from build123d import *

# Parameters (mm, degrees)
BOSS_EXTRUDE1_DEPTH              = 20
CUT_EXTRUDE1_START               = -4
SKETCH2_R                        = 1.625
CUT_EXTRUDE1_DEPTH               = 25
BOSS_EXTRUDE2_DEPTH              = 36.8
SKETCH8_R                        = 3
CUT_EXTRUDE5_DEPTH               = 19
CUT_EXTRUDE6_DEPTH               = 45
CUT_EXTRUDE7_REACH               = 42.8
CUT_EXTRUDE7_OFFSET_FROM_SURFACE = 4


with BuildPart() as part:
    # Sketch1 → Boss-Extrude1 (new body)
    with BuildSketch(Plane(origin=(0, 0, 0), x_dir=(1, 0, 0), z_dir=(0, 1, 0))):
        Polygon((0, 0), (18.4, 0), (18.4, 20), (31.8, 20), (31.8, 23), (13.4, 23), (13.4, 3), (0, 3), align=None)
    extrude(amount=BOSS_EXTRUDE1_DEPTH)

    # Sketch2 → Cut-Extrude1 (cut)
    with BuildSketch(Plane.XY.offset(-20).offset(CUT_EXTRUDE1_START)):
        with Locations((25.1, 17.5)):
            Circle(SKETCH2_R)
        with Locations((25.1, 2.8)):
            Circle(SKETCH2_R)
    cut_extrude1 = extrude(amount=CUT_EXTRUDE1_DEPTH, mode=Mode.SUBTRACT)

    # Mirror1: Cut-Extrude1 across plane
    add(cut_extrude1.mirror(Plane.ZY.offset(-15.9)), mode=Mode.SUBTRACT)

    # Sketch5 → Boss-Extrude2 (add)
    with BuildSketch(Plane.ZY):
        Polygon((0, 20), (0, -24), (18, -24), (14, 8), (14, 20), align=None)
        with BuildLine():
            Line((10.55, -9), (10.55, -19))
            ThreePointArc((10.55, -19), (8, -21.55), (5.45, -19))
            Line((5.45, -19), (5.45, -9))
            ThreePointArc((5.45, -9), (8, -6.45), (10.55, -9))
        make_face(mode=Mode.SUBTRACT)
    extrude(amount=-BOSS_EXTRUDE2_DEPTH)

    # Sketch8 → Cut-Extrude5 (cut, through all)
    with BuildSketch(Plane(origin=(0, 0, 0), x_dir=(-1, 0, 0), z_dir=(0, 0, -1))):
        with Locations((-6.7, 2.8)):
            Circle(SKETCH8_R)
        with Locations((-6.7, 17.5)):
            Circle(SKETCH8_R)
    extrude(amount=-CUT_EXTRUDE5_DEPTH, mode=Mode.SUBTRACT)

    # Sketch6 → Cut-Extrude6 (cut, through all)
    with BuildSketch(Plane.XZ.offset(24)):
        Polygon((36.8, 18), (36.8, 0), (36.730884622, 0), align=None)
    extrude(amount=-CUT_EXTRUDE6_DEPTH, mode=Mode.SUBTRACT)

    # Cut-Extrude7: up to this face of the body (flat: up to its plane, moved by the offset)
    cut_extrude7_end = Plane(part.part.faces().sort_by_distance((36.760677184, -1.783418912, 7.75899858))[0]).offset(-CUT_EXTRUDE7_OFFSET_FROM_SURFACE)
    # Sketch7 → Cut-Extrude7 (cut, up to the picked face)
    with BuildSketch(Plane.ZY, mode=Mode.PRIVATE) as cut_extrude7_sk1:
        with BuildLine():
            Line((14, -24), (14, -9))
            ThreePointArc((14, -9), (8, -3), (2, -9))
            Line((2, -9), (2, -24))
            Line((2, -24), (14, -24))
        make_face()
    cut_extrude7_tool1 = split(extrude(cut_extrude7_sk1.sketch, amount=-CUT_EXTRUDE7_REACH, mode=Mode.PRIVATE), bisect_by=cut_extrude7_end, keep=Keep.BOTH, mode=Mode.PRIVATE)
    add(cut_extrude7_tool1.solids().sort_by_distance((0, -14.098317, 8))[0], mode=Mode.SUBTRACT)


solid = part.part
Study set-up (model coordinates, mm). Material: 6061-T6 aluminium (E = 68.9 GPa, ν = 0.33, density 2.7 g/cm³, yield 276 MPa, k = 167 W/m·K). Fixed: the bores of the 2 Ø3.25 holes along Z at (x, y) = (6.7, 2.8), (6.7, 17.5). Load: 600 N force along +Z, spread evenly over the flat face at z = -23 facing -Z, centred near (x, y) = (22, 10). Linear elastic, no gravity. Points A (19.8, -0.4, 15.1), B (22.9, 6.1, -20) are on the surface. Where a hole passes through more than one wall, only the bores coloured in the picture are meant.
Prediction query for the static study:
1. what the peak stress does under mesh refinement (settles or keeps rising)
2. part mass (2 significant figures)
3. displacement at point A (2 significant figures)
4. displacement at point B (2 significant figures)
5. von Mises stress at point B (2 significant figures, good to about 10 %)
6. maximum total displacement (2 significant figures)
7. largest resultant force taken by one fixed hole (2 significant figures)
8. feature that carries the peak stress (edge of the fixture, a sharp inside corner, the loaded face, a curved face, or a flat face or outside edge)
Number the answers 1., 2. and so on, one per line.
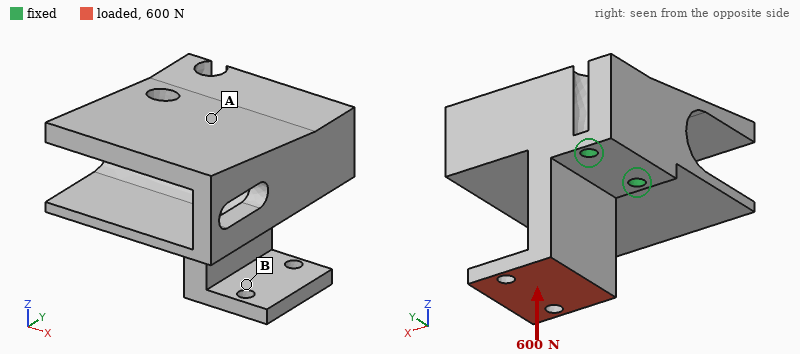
1. keeps rising
2. 54 g
3. 0.059 mm
4. 0.14 mm
5. 50 MPa
6. 0.26 mm
7. 310 N
8. edge of the fixture
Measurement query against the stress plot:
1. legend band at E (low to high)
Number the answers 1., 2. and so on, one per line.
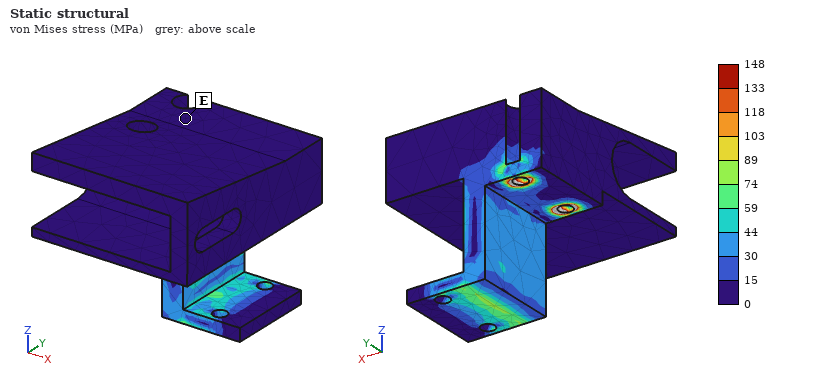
1. 0 to 15 MPa
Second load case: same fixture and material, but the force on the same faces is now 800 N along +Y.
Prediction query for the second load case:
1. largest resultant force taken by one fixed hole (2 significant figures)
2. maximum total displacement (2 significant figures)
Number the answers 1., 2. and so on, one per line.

1. 1.5 kN
2. 0.13 mm
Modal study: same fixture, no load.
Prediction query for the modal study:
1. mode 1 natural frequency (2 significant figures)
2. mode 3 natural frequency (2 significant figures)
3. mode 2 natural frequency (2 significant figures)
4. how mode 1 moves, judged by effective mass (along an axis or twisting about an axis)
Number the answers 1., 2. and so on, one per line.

1. 2000 Hz
2. 5200 Hz
3. 4500 Hz
4. along Z
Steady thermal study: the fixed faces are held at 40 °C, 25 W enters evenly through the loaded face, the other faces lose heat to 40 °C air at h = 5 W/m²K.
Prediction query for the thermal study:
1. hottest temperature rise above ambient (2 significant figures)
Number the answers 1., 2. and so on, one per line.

1. 56 K
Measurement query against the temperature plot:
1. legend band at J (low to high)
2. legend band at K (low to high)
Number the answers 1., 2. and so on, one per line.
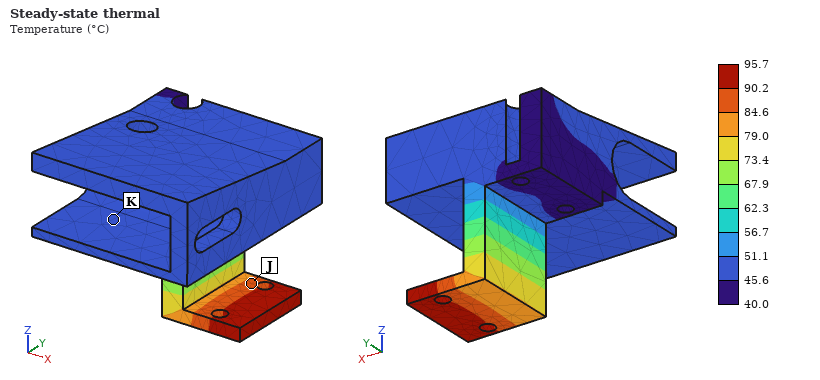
1. 84.6 to 90.2 °C
2. 45.6 to 51.1 °C
